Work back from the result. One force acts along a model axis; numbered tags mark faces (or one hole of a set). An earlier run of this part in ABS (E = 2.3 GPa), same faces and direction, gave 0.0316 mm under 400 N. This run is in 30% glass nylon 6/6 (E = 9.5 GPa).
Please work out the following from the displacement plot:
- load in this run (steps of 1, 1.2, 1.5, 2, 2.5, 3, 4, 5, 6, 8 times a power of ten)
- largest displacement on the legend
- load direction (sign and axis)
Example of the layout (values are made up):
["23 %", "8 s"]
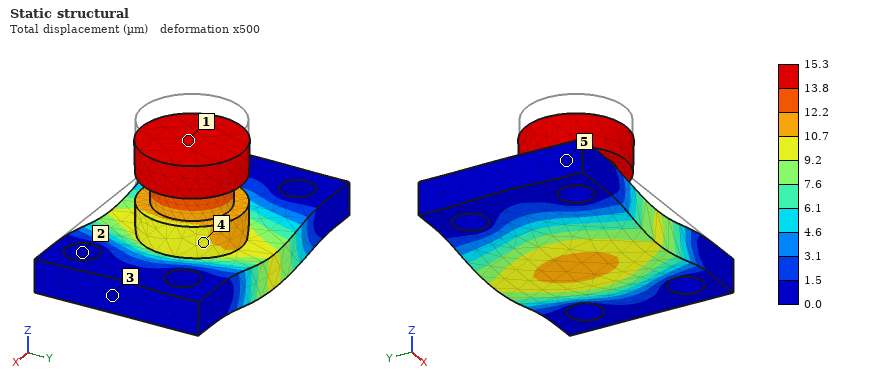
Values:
["800 N", "15.3 µm", "-Z"]
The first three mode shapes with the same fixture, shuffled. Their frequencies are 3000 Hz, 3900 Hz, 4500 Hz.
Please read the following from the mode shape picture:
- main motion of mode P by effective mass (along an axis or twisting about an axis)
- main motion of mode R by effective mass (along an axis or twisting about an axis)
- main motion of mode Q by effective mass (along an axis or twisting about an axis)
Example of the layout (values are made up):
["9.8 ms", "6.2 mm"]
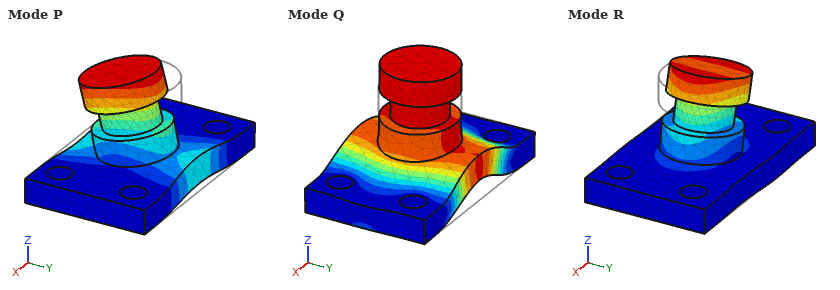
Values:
["along Y", "along X", "along Z"]
